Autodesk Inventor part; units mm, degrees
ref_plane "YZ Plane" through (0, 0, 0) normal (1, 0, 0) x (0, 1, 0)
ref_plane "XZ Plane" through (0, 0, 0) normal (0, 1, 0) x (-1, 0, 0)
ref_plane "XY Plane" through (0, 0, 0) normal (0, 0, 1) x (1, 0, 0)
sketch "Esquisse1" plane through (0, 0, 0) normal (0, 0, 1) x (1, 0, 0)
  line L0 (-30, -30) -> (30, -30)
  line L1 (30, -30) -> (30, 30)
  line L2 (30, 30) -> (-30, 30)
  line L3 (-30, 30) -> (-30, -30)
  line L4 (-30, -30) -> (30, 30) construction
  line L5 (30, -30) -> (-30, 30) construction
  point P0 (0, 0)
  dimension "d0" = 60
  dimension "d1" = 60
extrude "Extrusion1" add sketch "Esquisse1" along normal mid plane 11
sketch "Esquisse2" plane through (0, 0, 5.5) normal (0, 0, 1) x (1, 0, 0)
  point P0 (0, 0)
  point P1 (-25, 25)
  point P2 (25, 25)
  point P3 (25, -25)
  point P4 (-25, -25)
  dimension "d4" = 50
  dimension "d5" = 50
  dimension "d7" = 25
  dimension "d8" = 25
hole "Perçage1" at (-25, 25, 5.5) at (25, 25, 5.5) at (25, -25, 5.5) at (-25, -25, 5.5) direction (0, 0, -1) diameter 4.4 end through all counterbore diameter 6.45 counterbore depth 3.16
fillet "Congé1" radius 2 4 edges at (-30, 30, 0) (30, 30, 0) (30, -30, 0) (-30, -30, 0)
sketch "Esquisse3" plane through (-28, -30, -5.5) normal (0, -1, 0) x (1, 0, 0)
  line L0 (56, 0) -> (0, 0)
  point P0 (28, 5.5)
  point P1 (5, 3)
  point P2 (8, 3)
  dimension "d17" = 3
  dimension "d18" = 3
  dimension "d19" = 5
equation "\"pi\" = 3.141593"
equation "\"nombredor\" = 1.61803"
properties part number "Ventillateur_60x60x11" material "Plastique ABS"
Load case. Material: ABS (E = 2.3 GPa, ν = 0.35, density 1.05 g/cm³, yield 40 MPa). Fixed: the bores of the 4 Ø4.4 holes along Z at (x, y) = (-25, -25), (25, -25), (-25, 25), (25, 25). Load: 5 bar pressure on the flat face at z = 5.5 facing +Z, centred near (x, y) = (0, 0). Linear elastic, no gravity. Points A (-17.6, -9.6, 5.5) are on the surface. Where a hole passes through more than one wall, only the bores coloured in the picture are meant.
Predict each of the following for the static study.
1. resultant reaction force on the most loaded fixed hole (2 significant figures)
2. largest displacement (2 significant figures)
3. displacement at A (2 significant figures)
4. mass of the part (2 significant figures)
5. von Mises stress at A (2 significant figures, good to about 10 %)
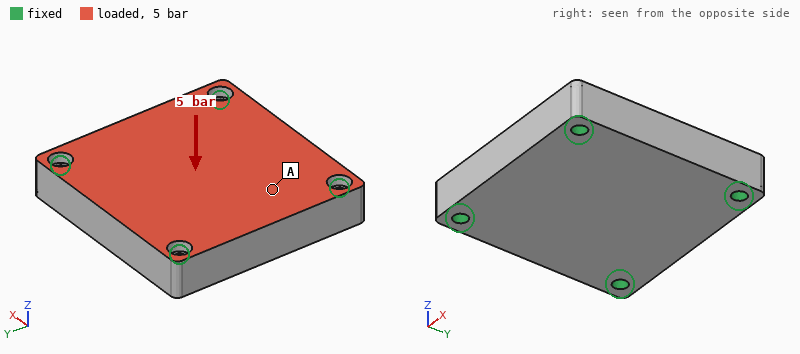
460 N
0.15 mm
0.10 mm
41 g
3.0 MPa
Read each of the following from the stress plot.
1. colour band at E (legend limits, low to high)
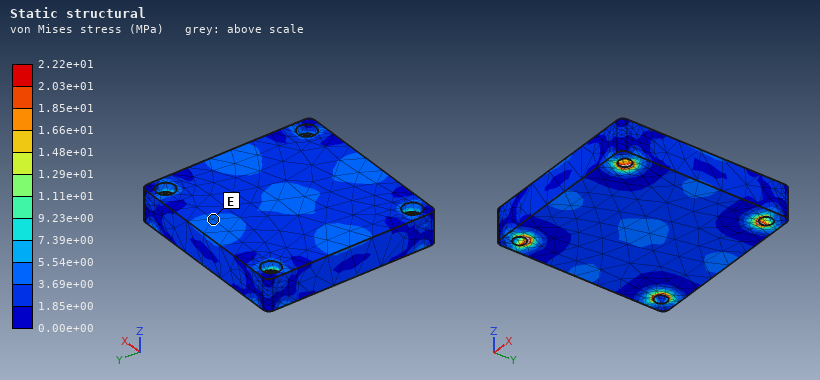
3.69e+00 to 5.54e+00 MPa
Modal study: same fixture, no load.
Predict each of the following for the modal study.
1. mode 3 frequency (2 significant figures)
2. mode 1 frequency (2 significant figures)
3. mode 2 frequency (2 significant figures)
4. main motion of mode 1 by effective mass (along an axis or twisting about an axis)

5100 Hz
3200 Hz
5100 Hz
along Z
